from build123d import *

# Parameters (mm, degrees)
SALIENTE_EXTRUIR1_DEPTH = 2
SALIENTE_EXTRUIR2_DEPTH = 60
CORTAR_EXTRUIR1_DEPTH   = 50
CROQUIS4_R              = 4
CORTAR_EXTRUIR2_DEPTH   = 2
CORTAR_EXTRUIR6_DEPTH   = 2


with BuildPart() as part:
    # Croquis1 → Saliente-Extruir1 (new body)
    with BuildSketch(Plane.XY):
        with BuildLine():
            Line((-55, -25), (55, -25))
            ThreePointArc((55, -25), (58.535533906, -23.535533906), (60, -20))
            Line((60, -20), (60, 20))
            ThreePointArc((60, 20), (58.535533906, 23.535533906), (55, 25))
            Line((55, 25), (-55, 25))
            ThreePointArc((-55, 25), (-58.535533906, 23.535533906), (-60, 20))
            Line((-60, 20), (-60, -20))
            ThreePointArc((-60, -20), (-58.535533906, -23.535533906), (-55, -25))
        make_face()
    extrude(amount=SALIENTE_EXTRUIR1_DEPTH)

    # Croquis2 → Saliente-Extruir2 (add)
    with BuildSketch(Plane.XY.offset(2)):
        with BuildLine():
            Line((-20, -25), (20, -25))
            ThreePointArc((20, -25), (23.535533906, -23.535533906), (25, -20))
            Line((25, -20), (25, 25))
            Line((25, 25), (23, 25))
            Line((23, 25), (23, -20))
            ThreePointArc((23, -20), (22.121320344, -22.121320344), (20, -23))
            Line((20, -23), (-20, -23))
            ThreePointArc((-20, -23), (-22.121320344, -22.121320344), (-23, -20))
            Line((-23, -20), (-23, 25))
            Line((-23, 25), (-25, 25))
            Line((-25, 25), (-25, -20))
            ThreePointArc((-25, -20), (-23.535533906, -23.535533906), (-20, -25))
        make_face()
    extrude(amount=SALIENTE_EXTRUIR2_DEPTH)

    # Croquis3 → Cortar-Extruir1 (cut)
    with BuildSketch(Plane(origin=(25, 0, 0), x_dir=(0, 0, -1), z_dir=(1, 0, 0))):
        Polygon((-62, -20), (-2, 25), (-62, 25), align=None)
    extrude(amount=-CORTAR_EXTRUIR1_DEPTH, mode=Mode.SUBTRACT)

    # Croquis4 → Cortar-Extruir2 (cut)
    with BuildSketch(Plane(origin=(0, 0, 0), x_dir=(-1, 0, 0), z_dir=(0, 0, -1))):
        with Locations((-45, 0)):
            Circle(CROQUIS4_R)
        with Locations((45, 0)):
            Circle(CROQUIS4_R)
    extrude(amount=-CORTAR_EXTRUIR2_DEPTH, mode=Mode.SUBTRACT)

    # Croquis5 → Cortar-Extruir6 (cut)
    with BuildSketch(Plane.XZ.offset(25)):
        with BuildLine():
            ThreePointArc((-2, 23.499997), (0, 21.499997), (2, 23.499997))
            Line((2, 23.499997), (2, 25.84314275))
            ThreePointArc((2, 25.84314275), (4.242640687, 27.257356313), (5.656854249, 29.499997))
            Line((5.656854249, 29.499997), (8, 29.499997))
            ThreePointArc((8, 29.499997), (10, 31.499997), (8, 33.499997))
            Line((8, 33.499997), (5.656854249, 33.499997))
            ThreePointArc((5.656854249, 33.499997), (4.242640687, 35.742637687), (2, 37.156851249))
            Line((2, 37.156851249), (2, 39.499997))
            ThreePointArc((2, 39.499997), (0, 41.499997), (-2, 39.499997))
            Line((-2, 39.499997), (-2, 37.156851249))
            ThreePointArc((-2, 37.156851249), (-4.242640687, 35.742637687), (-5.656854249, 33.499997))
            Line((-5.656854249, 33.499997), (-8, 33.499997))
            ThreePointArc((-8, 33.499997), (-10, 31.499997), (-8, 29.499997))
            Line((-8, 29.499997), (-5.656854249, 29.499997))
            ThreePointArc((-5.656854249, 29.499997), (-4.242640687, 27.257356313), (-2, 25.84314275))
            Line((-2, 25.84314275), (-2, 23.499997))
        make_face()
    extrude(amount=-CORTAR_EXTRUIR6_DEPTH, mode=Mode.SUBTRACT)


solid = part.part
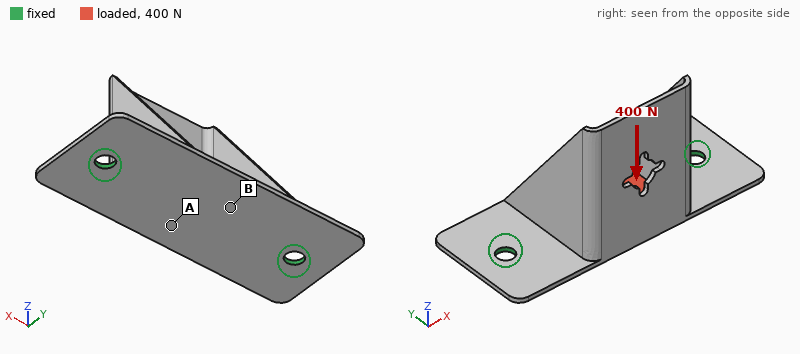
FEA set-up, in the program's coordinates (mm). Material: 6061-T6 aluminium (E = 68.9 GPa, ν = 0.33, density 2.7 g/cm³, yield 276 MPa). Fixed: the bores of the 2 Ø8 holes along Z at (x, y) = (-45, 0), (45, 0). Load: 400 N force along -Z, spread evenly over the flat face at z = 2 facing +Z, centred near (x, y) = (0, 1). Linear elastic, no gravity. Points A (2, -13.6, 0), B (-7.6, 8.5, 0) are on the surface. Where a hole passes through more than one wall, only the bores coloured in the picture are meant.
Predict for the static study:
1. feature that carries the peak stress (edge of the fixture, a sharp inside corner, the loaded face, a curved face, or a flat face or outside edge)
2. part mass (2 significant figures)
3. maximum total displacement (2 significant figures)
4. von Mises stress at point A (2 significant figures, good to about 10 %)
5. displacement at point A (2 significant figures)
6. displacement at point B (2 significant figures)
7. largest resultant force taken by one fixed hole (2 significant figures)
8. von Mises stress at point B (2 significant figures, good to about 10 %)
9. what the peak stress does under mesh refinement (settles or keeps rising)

edge of the fixture
62 g
0.42 mm
14 MPa
0.15 mm
0.30 mm
210 N
39 MPa
keeps rising
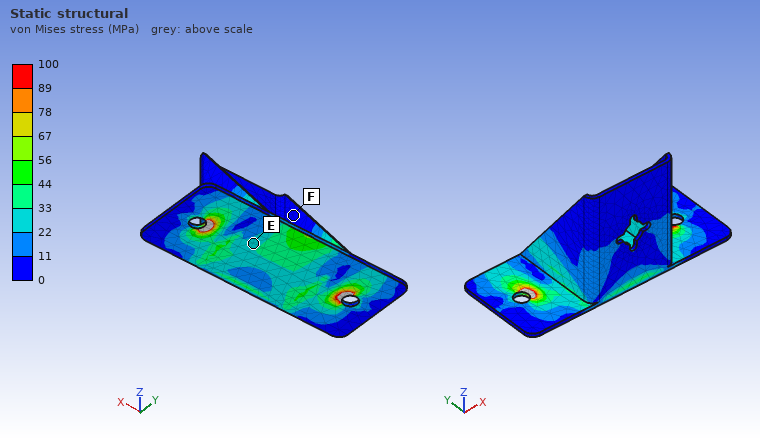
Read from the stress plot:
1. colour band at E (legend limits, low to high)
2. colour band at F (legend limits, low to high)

22 to 33 MPa
0 to 11 MPa
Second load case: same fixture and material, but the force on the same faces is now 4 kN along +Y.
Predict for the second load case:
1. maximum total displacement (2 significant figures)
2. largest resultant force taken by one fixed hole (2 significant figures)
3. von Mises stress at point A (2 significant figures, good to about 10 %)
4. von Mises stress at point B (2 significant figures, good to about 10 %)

0.59 mm
2.0 kN
24 MPa
27 MPa
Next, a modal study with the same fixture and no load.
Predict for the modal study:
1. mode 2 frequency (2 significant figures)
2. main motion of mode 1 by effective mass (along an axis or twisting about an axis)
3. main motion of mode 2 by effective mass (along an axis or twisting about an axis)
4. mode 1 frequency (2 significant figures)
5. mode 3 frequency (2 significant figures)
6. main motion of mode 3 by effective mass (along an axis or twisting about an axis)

990 Hz
along Y
along X
540 Hz
1300 Hz
along Z
